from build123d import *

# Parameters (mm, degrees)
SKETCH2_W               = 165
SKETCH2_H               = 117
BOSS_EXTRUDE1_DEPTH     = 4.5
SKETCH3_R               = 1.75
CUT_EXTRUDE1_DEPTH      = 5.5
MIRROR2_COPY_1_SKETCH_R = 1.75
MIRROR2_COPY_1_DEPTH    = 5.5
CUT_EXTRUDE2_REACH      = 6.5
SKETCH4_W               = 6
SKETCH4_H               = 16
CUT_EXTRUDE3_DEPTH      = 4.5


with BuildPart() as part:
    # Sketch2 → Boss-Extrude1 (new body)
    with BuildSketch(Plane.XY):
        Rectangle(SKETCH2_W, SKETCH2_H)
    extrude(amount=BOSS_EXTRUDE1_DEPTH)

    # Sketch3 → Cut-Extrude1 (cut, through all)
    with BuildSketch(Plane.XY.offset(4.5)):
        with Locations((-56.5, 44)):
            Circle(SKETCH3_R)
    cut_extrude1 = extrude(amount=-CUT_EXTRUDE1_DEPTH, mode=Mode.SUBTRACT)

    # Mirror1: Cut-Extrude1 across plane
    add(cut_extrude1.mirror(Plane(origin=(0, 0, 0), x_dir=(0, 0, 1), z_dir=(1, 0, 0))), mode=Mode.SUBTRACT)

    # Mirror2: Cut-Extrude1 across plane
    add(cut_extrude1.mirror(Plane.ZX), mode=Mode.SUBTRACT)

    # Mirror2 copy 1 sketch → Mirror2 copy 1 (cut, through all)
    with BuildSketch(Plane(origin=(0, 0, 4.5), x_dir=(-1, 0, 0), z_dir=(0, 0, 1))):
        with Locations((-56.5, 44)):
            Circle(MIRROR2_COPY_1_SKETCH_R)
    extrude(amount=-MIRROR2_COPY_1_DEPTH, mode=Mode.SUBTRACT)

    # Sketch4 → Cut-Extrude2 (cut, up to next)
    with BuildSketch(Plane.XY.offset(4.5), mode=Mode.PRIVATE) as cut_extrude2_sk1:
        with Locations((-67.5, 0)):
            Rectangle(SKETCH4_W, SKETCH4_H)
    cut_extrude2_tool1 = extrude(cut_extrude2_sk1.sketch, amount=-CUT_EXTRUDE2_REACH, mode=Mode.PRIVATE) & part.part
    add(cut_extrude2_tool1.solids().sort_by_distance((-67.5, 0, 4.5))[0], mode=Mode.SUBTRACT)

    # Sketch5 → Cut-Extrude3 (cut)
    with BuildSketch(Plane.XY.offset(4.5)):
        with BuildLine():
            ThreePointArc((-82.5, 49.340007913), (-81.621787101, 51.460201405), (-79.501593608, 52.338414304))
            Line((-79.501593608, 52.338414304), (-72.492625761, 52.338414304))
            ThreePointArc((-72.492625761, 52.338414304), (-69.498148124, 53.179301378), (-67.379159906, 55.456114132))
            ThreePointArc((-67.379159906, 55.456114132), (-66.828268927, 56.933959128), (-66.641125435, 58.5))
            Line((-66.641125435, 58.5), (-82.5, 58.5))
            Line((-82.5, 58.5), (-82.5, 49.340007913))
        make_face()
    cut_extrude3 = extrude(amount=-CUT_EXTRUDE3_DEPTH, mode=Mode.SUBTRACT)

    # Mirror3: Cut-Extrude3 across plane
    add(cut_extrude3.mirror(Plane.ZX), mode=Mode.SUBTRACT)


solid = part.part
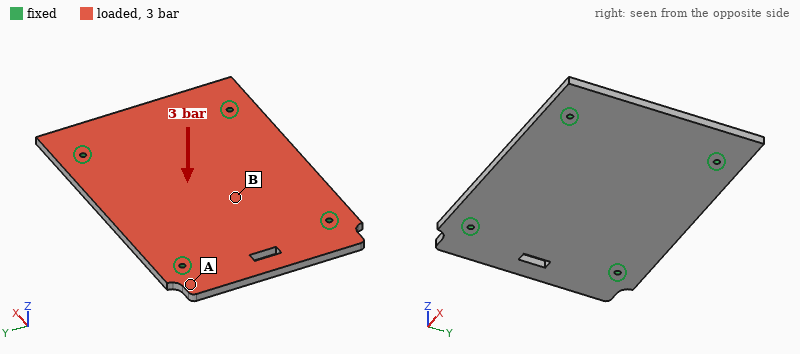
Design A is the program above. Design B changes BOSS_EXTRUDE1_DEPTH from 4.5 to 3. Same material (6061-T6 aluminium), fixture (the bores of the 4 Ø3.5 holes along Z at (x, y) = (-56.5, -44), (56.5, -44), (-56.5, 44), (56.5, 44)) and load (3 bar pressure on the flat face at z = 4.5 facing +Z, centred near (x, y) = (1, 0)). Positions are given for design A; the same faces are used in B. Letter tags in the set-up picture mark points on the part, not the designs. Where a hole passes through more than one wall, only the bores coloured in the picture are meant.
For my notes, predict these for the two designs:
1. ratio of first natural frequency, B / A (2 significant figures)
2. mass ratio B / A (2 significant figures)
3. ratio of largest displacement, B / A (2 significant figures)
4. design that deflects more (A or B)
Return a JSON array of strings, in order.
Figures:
["0.69", "0.67", "3.2", "B"]
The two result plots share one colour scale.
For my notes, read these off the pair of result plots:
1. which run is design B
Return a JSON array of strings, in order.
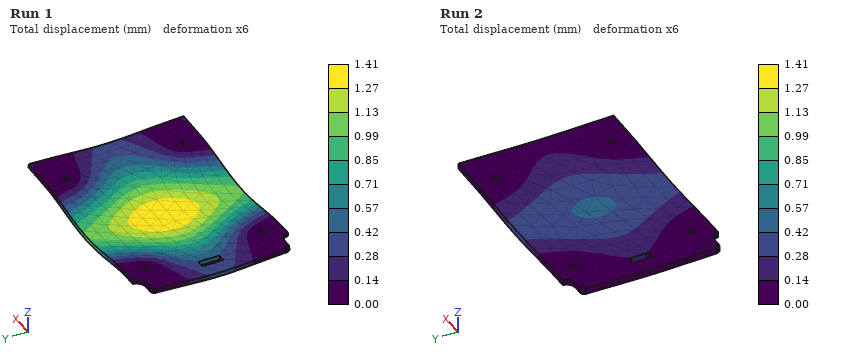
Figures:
["Run 1"]
